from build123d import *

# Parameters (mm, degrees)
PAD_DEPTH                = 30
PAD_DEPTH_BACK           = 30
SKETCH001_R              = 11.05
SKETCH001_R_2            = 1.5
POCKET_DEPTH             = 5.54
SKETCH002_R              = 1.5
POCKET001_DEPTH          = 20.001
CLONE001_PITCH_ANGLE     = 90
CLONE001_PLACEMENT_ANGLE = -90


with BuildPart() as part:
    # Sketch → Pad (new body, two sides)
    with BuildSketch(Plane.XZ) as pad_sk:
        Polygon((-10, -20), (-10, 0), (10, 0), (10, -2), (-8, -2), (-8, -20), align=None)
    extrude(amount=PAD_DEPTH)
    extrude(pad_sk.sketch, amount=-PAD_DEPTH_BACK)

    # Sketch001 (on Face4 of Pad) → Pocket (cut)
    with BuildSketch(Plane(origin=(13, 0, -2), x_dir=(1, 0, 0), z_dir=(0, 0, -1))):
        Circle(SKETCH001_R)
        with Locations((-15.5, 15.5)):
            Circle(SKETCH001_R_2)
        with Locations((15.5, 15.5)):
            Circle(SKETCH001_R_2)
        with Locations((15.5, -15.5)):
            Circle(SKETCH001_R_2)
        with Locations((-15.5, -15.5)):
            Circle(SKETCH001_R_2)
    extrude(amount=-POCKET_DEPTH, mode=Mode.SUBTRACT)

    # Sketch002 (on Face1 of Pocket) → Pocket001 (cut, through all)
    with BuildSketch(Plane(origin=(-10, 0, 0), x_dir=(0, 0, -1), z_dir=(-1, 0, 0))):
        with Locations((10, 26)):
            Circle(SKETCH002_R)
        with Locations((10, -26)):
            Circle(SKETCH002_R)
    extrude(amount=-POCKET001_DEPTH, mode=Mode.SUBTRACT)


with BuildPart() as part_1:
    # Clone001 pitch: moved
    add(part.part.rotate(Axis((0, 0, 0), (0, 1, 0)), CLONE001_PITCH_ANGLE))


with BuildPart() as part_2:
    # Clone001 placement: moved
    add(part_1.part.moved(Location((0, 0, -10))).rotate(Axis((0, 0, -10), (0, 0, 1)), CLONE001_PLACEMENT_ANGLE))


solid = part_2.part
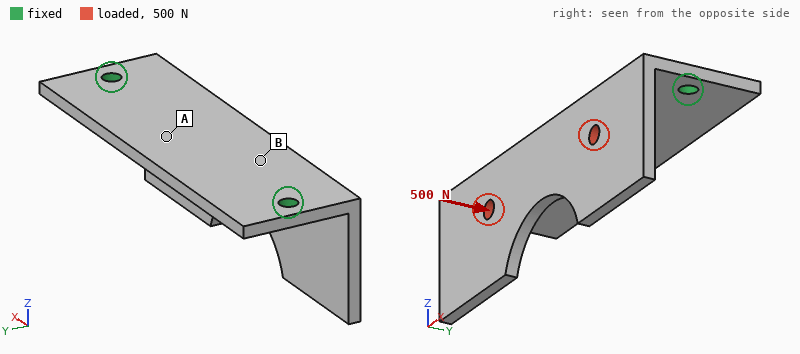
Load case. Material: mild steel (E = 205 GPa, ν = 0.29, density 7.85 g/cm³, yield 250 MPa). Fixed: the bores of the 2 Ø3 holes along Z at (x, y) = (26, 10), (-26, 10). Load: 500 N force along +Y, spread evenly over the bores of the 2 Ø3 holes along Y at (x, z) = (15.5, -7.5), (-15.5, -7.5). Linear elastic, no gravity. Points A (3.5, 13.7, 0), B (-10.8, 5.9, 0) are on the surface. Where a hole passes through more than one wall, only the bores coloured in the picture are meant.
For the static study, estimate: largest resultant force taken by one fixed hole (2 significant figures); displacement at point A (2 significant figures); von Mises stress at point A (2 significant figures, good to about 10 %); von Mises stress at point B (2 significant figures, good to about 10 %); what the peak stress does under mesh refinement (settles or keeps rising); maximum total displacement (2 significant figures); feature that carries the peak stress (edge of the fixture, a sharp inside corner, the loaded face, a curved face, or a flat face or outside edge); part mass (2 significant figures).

250 N
0.024 mm
26 MPa
54 MPa
keeps rising
0.12 mm
edge of the fixture
33 g
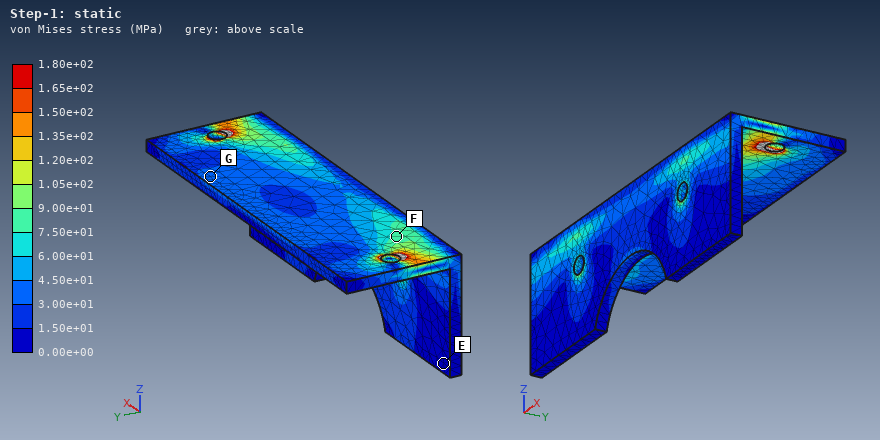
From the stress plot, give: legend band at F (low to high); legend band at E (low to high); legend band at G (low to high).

7.50e+01 to 9.00e+01 MPa
0.00e+00 to 1.50e+01 MPa
3.00e+01 to 4.50e+01 MPa
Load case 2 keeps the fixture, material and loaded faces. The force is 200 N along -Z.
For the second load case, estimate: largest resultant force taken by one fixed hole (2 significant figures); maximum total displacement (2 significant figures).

110 N
35 µm
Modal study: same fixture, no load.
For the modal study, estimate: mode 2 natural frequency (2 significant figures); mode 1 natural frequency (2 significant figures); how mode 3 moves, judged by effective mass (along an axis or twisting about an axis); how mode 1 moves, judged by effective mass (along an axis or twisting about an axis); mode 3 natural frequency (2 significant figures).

3600 Hz
2400 Hz
along Z
along Y
5000 Hz
